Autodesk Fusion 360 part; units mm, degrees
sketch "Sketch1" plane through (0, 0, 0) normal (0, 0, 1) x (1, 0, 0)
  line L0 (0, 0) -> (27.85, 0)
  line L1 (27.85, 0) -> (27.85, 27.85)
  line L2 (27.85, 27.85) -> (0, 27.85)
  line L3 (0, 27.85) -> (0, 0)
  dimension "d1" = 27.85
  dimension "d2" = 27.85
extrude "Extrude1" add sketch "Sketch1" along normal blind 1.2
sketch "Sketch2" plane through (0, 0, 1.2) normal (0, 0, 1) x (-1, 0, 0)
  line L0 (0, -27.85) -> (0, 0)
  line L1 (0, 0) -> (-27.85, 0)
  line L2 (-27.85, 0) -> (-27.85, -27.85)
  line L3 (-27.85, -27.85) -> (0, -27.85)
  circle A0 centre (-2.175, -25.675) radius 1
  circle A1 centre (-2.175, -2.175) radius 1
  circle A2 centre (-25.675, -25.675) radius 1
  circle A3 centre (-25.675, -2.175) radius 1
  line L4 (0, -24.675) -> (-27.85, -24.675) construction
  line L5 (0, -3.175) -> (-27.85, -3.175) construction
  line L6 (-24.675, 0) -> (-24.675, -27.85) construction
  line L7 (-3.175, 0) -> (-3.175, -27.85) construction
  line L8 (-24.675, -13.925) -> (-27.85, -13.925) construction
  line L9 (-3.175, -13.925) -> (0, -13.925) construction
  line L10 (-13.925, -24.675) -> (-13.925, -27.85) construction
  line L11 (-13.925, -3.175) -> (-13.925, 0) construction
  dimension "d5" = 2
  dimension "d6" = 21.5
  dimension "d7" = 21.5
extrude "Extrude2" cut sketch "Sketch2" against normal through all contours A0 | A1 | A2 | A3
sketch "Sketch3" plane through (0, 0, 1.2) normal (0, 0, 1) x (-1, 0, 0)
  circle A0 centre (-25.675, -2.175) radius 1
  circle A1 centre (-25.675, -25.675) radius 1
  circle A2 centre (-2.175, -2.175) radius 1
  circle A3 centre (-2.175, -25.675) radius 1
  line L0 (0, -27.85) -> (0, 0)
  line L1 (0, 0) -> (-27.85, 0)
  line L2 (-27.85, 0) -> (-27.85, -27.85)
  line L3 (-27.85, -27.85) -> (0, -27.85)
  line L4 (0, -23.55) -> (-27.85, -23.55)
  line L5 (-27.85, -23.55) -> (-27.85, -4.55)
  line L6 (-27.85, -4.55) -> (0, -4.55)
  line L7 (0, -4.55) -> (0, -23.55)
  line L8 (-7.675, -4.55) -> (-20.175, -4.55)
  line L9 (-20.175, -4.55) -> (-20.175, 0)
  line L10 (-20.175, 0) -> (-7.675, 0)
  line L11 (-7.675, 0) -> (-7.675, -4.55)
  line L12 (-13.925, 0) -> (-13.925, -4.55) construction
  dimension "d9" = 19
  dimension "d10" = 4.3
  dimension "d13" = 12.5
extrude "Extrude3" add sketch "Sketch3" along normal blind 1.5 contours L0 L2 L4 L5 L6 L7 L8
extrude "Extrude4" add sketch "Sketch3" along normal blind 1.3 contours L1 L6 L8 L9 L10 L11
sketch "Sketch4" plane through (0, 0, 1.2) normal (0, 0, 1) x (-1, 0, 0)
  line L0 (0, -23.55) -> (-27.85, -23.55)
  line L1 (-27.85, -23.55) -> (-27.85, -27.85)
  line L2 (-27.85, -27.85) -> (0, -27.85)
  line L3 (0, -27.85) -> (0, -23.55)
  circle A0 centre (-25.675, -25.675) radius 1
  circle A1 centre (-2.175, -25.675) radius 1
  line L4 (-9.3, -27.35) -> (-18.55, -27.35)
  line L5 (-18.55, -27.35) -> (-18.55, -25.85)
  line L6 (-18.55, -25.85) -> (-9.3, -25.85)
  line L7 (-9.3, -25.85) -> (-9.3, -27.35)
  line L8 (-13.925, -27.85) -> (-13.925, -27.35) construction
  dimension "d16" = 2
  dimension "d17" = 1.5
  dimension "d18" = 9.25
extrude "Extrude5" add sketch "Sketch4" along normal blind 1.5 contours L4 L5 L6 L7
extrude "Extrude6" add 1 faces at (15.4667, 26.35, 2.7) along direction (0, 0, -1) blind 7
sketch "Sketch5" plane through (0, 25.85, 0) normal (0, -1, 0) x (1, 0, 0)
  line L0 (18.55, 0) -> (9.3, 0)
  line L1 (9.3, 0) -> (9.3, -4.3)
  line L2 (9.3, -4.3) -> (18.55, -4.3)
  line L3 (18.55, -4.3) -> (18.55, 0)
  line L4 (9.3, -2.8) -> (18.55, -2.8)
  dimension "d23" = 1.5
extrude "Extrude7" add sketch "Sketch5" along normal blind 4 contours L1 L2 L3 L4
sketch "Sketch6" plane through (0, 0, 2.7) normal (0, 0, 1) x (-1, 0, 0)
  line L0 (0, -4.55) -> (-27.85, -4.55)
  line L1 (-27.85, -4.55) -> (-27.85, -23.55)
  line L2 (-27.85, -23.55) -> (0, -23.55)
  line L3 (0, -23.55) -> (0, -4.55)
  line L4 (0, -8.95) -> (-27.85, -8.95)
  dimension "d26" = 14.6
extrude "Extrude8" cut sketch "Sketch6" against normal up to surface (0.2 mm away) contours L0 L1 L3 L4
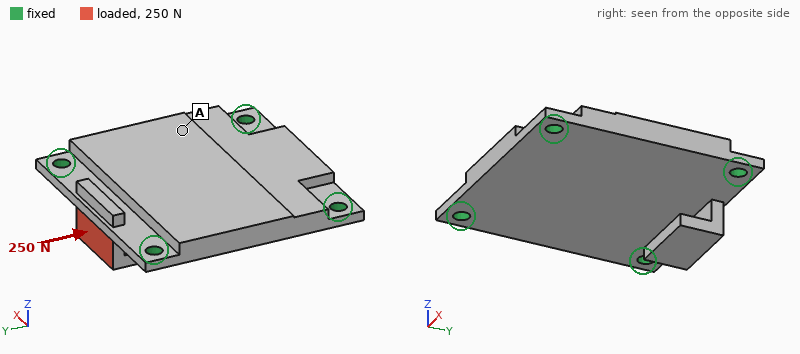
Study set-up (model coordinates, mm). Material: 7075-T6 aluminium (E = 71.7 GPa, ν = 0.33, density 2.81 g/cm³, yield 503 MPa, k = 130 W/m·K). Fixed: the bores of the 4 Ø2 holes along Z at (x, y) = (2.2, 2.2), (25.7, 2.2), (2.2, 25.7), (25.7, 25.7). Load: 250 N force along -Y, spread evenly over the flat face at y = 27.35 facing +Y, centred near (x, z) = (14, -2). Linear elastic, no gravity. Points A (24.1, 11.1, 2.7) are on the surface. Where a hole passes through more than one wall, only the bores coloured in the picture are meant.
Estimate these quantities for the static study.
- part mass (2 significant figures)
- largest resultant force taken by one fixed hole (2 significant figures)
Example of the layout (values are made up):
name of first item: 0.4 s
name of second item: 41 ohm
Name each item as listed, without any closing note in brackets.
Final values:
part mass: 5.3 g
largest resultant force taken by one fixed hole: 100 N
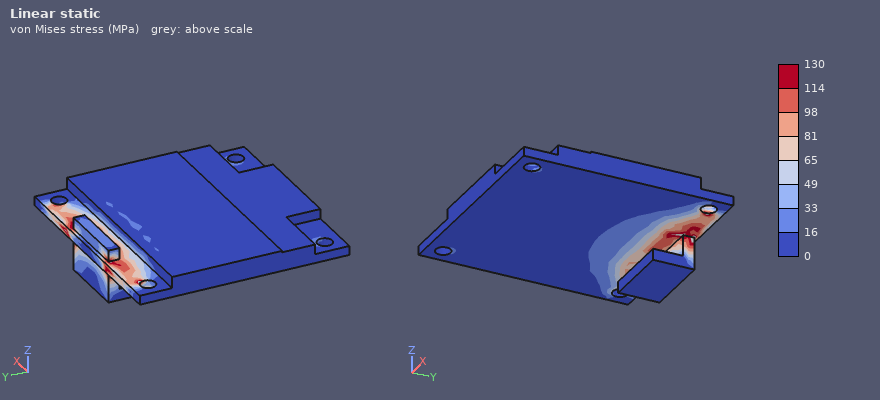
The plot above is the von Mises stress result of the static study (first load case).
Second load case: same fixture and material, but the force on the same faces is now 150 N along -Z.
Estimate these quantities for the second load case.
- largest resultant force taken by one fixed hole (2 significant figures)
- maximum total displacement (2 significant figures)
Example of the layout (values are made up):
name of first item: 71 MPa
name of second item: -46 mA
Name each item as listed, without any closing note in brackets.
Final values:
largest resultant force taken by one fixed hole: 86 N
maximum total displacement: 55 µm
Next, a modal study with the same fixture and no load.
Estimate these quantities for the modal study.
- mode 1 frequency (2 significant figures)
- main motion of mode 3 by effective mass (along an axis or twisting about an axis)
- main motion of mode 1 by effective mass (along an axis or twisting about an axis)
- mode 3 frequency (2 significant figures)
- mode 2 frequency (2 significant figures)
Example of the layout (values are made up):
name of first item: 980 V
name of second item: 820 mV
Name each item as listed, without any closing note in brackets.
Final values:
mode 1 frequency: 11 kHz
main motion of mode 3 by effective mass: twisting about X
main motion of mode 1 by effective mass: along Z
mode 3 frequency: 17 kHz
mode 2 frequency: 13 kHz
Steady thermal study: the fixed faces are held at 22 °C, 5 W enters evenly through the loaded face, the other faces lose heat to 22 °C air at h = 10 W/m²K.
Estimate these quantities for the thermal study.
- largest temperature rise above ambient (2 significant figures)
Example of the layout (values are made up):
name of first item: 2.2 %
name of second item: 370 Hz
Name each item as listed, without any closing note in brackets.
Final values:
largest temperature rise above ambient: 21 K
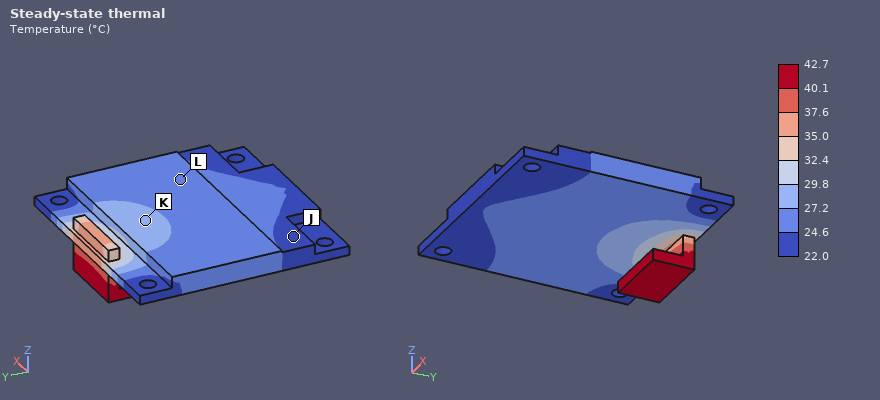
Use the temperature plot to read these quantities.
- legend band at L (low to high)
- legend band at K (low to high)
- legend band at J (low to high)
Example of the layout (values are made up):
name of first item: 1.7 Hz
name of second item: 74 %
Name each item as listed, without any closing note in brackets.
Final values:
legend band at L: 24.6 to 27.2 °C
legend band at K: 27.2 to 29.8 °C
legend band at J: 22.0 to 24.6 °C
